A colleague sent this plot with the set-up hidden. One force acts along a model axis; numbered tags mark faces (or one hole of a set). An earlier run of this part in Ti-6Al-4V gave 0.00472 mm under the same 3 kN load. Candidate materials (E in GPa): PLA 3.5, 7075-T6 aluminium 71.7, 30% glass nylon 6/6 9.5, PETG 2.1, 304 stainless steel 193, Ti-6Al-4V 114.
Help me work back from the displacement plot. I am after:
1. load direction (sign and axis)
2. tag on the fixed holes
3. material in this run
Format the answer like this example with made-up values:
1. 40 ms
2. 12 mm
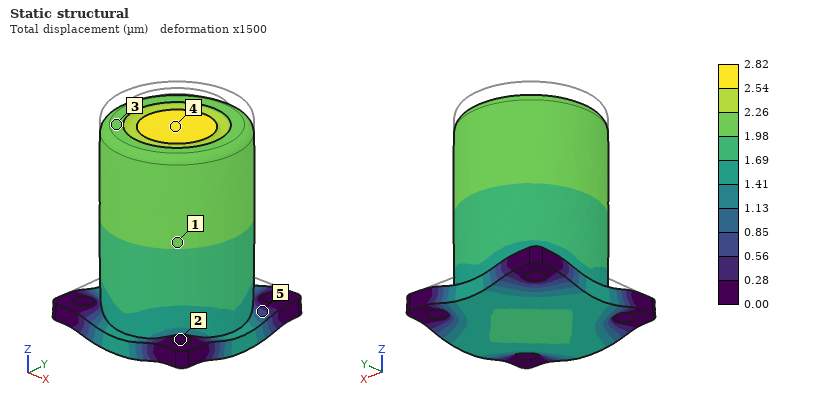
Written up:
1. -Z
2. 2
3. 304 stainless steel
